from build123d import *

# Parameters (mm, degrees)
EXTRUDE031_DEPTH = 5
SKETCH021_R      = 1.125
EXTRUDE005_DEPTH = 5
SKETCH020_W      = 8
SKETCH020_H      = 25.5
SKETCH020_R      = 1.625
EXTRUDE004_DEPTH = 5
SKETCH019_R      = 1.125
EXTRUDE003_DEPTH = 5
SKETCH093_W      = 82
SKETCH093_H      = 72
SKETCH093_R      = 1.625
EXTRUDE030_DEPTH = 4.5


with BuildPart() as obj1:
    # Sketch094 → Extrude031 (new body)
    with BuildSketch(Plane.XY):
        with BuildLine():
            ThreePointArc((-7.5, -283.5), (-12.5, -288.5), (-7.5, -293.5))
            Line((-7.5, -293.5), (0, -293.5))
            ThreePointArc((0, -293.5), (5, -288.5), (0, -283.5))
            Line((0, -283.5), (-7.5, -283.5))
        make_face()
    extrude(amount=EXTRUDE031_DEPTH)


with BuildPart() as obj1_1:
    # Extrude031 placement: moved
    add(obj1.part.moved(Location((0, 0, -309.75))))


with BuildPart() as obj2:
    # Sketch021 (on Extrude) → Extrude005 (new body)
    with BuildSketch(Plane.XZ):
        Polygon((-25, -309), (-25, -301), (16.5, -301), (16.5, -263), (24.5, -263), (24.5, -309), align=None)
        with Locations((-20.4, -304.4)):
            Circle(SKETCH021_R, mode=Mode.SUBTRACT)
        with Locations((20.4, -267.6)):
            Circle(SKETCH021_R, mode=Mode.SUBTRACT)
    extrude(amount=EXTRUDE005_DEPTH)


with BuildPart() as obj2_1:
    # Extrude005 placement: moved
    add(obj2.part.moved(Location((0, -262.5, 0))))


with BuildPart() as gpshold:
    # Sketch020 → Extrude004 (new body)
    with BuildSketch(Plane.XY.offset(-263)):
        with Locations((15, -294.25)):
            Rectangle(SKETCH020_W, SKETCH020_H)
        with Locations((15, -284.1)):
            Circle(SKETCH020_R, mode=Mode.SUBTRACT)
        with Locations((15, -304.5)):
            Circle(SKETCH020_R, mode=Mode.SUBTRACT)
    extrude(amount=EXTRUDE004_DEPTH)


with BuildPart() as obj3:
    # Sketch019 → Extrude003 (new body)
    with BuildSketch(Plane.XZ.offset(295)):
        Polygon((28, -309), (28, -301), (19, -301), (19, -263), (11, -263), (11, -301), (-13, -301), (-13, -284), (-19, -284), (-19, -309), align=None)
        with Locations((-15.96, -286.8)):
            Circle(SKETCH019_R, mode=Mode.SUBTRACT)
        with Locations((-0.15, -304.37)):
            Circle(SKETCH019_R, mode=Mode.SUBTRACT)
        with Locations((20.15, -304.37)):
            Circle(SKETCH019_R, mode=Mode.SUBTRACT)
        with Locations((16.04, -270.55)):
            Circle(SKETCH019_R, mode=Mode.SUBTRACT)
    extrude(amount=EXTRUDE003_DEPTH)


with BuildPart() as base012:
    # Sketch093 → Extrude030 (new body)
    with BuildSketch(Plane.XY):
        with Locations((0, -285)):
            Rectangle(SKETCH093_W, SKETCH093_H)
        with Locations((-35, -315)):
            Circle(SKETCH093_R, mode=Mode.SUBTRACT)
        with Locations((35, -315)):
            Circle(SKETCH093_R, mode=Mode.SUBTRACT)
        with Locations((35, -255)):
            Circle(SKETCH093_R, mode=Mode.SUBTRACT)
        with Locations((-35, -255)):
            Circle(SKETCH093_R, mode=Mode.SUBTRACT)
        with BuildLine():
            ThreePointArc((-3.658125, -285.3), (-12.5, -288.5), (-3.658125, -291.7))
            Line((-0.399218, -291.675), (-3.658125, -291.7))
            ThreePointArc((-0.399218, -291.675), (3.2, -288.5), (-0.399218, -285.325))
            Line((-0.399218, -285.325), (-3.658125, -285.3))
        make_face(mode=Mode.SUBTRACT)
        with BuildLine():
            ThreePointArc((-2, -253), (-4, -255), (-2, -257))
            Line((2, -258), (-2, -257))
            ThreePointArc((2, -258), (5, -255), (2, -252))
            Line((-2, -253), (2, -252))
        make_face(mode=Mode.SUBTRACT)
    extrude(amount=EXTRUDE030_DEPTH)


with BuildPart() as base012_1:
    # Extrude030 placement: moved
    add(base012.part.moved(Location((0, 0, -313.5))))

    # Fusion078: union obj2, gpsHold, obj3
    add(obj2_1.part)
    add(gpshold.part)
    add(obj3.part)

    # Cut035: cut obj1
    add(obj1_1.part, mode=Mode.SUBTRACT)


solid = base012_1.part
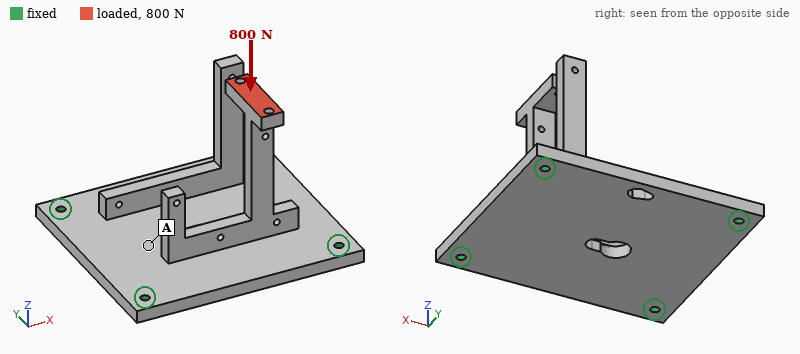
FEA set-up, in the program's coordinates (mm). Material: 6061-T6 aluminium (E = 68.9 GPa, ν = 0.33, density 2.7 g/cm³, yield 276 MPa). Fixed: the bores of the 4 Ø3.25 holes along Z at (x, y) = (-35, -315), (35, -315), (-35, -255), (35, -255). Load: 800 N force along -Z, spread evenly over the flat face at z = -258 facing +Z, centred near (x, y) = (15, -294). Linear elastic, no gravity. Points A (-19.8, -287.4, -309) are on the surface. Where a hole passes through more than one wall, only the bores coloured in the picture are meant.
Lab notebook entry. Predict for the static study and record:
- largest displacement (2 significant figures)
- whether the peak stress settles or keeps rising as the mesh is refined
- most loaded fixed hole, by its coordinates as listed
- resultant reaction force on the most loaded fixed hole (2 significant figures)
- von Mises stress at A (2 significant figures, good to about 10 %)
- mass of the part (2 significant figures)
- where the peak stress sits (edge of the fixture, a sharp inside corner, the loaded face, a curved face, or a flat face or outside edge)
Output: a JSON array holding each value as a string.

["0.76 mm", "keeps rising", "(35, -315)", "410 N", "14 MPa", "92 g", "a sharp inside corner"]
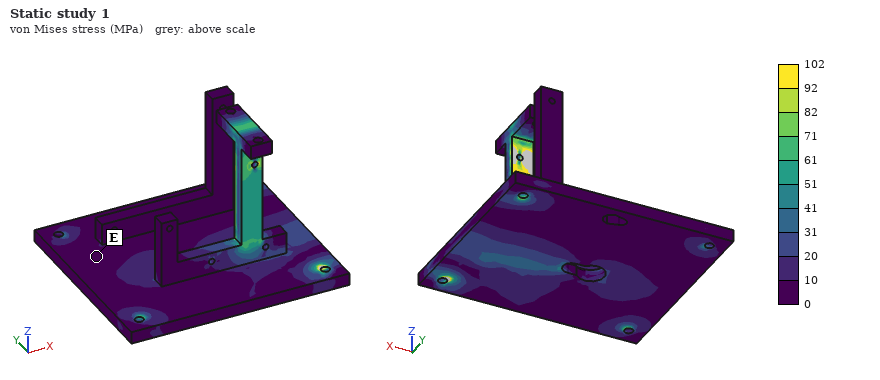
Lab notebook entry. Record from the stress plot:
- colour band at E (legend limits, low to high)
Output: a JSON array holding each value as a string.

["0 to 10 MPa"]
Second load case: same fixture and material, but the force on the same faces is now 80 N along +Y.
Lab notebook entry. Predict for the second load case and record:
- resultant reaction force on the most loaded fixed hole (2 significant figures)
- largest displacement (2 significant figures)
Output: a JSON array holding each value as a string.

["70 N", "0.65 mm"]
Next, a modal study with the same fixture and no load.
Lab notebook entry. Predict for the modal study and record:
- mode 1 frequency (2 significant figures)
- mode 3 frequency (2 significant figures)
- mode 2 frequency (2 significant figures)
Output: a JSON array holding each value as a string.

["1000 Hz", "1900 Hz", "1800 Hz"]
